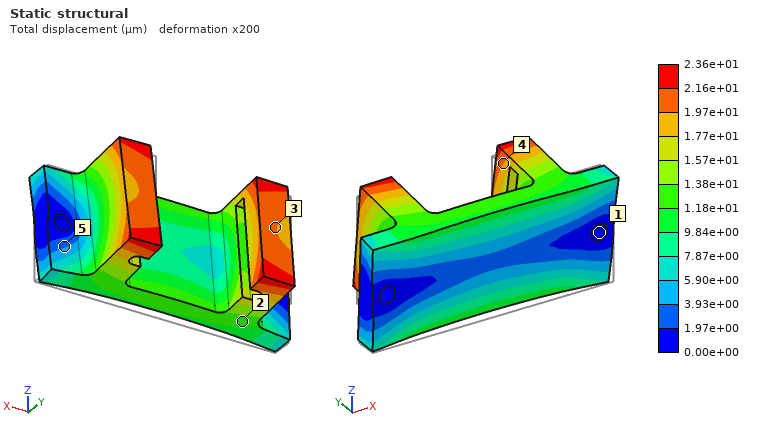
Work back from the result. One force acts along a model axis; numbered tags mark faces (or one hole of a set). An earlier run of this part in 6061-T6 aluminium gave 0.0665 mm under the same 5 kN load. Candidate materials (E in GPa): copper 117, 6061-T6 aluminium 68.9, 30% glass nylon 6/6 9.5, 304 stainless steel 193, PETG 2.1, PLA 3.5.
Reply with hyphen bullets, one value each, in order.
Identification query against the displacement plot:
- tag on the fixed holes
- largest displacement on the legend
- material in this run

- 1
- 2.36e+01 µm
- 304 stainless steel
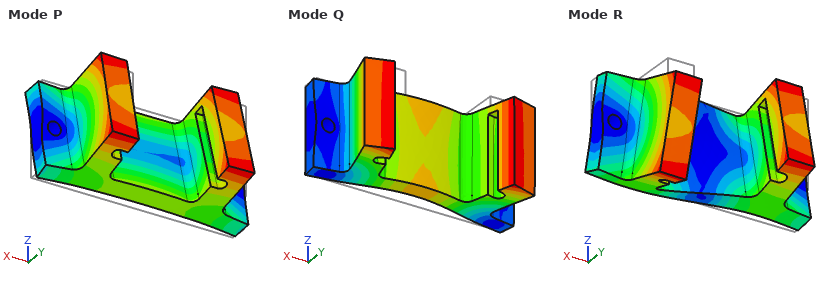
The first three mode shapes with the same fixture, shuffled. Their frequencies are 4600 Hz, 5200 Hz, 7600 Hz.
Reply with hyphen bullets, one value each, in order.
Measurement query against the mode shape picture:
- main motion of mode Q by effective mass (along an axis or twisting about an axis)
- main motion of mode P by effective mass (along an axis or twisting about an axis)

- along Y
- along Z
